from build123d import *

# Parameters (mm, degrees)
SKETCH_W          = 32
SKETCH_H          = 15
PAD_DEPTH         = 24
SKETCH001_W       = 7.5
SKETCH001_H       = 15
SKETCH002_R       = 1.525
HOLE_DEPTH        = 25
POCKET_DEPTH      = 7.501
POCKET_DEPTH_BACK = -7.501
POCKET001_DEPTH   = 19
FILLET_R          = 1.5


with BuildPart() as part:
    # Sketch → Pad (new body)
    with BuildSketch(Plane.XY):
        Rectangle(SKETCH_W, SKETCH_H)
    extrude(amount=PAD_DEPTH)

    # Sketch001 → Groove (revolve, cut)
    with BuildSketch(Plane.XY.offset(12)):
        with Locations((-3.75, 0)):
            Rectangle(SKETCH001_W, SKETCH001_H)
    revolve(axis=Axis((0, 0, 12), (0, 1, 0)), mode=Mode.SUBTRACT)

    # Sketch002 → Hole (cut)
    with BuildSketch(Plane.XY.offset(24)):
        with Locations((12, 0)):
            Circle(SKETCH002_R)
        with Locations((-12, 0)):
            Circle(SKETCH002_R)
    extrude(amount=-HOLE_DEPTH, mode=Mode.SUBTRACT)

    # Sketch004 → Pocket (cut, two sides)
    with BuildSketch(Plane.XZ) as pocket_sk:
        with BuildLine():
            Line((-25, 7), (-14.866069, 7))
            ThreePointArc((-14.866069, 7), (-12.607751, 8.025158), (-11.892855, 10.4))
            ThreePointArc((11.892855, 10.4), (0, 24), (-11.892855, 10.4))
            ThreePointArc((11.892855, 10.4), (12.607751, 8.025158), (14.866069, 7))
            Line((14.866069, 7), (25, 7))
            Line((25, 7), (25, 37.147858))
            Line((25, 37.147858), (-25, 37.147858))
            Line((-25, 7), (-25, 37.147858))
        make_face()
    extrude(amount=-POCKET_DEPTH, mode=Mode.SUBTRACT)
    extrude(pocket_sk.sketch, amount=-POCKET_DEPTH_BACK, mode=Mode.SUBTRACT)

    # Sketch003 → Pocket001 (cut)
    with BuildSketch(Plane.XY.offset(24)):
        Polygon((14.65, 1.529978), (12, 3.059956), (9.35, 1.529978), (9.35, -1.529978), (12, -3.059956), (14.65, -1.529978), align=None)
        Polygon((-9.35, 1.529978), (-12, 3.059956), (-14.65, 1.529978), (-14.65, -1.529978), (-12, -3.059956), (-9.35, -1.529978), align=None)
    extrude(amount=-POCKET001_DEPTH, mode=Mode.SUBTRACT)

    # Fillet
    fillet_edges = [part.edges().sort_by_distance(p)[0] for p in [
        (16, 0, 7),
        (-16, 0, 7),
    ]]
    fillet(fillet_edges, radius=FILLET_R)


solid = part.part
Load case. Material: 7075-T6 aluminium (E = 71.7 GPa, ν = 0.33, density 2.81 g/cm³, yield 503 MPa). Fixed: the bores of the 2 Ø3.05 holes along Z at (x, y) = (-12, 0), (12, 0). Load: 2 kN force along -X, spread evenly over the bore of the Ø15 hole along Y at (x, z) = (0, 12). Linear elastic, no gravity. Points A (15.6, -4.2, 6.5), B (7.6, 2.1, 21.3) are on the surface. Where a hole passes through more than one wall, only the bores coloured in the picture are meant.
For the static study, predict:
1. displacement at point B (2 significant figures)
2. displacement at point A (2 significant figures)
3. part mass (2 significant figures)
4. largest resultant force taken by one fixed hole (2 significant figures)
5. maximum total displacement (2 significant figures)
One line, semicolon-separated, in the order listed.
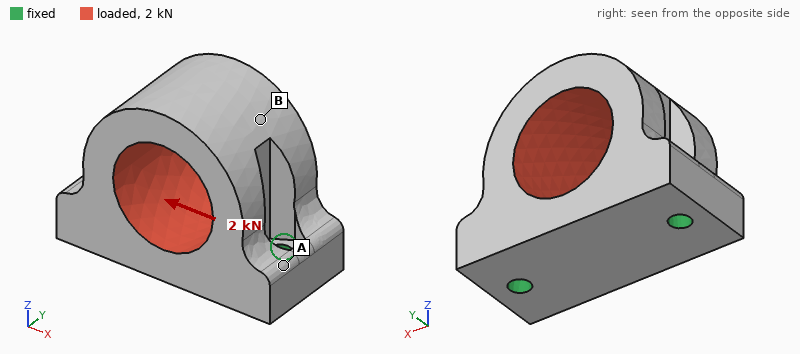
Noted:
20 µm; 4.0 µm; 15 g; 1.2 kN; 20 µm
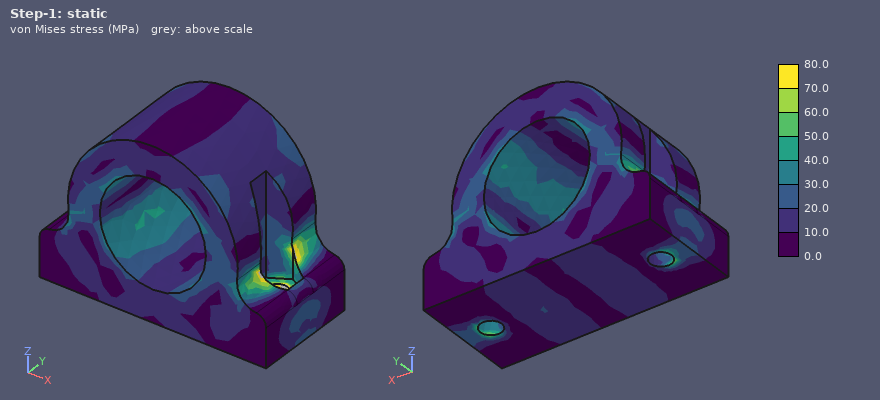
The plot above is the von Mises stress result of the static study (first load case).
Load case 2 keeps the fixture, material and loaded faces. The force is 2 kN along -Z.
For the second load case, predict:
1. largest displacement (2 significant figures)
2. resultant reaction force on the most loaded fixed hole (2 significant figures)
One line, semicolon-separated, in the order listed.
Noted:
6.1 µm; 1.0 kN
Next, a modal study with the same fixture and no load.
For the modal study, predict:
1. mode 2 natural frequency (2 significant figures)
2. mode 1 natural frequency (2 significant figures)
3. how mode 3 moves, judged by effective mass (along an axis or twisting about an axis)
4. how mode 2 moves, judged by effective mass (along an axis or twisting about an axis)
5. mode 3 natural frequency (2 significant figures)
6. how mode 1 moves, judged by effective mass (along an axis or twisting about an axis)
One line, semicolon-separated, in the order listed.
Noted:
16 kHz; 9900 Hz; twisting about Z; along X; 22 kHz; along Y
